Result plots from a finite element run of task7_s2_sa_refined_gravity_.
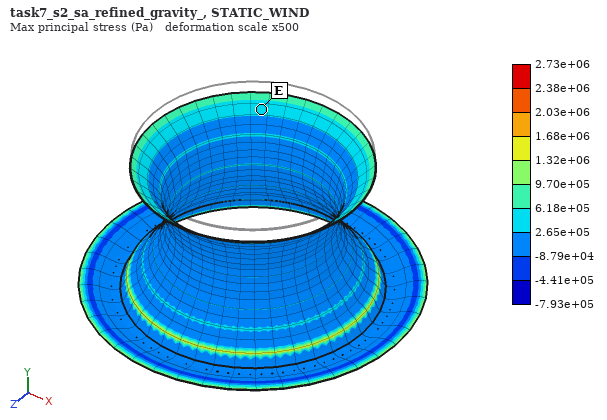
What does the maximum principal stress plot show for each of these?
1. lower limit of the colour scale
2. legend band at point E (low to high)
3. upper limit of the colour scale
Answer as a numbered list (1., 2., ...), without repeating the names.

1. -7.93e+05 Pa
2. 2.65e+05 to 6.18e+05 Pa
3. 2.73e+06 Pa
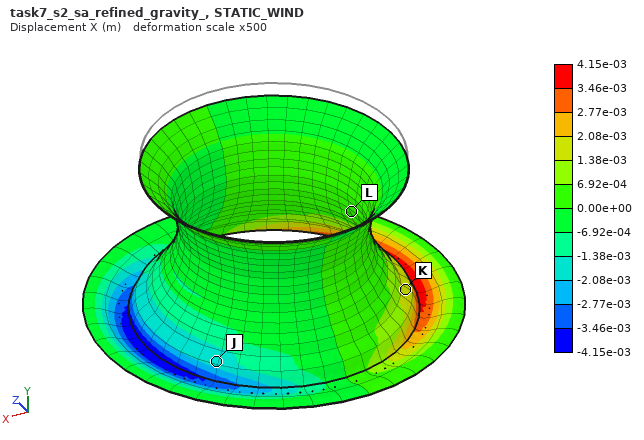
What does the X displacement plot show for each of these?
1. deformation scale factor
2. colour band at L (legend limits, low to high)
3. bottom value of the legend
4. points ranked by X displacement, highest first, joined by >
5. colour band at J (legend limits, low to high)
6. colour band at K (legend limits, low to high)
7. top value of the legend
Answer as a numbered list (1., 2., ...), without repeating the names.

1. 500
2. 0.00e+00 to 6.92e-04 m
3. -4.15e-03 m
4. K > L > J
5. -2.08e-03 to -1.38e-03 m
6. 1.38e-03 to 2.08e-03 m
7. 4.15e-03 m
